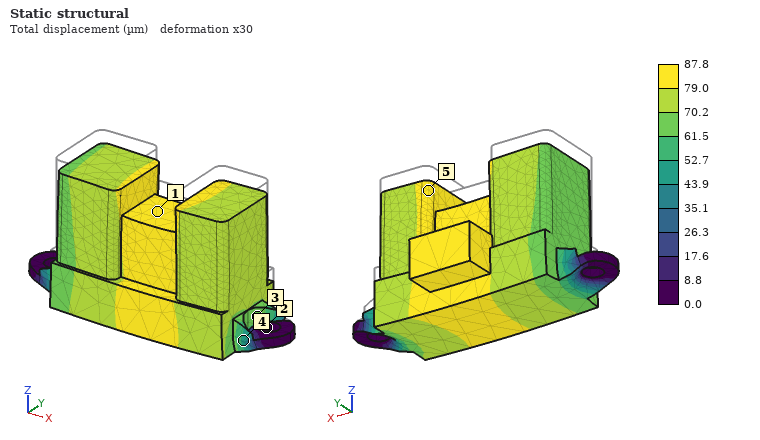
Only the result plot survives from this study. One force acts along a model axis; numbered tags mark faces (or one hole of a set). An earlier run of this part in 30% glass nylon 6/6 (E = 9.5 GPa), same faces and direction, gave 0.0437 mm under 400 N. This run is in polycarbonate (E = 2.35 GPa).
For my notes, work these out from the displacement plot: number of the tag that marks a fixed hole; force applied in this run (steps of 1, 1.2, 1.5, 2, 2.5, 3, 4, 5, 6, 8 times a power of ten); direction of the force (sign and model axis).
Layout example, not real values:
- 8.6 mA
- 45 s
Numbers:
- 2
- 200 N
- -Z
